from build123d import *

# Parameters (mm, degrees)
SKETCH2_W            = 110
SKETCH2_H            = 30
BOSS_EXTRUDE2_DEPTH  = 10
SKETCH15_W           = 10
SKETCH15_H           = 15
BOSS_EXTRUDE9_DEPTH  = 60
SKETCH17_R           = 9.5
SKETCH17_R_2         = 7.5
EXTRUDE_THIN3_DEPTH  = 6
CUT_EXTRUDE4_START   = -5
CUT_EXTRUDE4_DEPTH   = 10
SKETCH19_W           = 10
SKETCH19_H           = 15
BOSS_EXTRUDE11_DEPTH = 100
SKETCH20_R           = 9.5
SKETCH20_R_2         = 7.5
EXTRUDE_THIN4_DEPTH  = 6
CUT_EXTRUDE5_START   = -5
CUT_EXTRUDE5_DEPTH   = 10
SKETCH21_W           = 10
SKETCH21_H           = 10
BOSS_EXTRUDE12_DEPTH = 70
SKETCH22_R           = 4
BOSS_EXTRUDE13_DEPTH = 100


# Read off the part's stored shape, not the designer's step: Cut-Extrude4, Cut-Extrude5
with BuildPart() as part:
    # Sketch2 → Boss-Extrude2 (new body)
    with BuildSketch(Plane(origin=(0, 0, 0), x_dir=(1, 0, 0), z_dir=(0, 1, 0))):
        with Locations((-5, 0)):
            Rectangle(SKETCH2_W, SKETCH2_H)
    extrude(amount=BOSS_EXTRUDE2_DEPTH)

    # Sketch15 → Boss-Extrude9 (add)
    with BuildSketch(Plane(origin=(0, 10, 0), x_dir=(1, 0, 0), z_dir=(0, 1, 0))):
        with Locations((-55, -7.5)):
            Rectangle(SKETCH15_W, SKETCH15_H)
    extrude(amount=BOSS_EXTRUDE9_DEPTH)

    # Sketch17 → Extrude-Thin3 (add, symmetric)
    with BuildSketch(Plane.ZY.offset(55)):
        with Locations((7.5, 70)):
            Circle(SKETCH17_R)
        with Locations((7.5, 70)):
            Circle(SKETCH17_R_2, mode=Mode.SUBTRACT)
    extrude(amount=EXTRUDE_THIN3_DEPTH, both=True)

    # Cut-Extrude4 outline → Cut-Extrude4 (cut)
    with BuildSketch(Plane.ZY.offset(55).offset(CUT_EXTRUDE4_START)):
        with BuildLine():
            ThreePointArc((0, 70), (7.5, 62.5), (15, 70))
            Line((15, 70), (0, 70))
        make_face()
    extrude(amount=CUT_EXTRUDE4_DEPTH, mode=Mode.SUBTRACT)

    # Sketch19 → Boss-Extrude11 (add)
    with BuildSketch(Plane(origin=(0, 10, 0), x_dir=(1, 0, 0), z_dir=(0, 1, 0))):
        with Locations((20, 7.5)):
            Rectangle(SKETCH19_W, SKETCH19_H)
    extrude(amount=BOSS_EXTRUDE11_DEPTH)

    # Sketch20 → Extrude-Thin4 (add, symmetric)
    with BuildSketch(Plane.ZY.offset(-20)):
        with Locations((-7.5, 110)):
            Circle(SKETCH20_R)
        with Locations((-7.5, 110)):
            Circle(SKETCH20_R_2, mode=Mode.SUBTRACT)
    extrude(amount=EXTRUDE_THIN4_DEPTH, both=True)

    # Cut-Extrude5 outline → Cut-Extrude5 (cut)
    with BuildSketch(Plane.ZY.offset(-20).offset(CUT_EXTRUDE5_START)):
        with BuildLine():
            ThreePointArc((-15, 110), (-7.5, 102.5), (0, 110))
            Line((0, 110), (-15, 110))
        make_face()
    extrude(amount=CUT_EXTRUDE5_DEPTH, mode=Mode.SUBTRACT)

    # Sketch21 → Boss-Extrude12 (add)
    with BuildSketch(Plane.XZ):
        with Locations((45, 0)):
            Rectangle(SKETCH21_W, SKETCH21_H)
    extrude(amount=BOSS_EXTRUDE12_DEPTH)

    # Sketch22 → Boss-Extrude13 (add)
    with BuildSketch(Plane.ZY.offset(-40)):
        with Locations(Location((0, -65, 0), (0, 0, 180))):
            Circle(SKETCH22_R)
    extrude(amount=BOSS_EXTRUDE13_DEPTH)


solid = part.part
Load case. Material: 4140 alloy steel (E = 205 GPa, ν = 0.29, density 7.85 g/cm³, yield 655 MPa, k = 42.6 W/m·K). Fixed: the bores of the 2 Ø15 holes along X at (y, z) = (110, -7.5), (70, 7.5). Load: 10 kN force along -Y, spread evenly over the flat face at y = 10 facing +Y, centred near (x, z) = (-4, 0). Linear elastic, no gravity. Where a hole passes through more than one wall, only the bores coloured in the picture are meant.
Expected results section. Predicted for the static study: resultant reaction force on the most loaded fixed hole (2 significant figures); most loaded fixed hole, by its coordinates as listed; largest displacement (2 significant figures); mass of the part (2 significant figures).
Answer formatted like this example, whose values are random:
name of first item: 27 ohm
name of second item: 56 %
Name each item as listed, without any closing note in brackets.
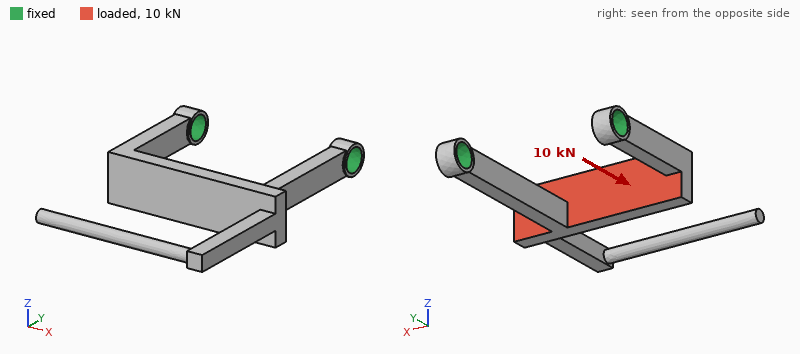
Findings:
resultant reaction force on the most loaded fixed hole: 6.8 kN
most loaded fixed hole, by its coordinates as listed: (110, -7.5)
largest displacement: 0.43 mm
mass of the part: 540 g
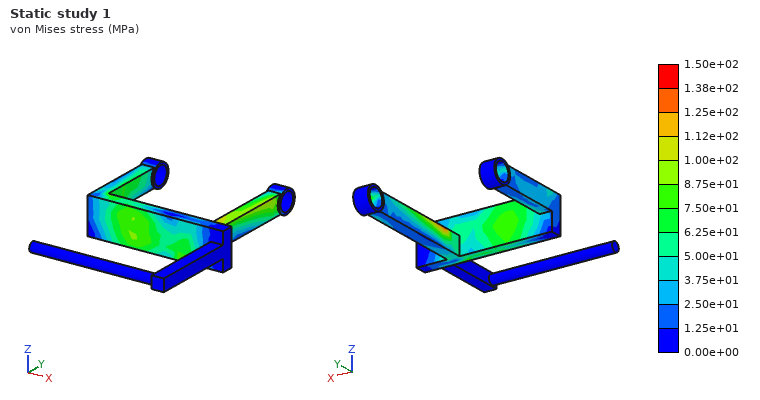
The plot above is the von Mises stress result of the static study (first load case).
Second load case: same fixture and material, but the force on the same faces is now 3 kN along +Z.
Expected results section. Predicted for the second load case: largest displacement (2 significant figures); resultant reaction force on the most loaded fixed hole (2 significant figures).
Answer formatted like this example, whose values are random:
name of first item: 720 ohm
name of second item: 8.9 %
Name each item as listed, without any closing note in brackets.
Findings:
largest displacement: 1.4 mm
resultant reaction force on the most loaded fixed hole: 1.5 kN
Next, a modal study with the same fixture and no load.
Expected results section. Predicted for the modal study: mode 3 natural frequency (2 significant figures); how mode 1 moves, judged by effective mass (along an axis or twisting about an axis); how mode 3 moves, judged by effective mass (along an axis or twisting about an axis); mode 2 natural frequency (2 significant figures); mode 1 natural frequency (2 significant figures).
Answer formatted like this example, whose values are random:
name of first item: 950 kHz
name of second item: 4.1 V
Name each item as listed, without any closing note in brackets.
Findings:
mode 3 natural frequency: 490 Hz
how mode 1 moves, judged by effective mass: along Z
how mode 3 moves, judged by effective mass: along Z
mode 2 natural frequency: 380 Hz
mode 1 natural frequency: 320 Hz
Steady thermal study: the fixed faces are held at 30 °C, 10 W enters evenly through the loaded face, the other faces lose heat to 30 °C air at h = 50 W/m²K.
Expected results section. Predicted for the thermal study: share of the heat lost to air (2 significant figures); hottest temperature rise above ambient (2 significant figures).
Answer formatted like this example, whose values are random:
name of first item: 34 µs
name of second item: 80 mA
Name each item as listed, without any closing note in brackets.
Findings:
share of the heat lost to air: 81 %
hottest temperature rise above ambient: 18 K
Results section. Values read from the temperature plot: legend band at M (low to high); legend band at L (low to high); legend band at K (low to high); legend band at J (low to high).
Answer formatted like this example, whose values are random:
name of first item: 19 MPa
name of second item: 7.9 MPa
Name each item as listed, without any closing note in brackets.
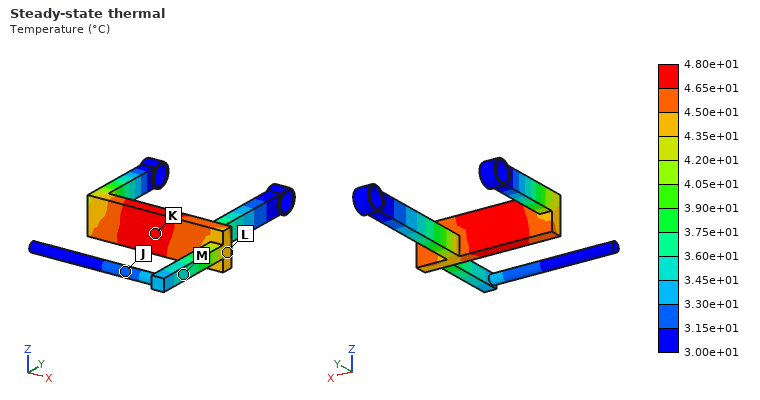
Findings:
legend band at M: 3.45e+01 to 3.60e+01 °C
legend band at L: 4.35e+01 to 4.50e+01 °C
legend band at K: 4.65e+01 to 4.80e+01 °C
legend band at J: 3.15e+01 to 3.30e+01 °C
